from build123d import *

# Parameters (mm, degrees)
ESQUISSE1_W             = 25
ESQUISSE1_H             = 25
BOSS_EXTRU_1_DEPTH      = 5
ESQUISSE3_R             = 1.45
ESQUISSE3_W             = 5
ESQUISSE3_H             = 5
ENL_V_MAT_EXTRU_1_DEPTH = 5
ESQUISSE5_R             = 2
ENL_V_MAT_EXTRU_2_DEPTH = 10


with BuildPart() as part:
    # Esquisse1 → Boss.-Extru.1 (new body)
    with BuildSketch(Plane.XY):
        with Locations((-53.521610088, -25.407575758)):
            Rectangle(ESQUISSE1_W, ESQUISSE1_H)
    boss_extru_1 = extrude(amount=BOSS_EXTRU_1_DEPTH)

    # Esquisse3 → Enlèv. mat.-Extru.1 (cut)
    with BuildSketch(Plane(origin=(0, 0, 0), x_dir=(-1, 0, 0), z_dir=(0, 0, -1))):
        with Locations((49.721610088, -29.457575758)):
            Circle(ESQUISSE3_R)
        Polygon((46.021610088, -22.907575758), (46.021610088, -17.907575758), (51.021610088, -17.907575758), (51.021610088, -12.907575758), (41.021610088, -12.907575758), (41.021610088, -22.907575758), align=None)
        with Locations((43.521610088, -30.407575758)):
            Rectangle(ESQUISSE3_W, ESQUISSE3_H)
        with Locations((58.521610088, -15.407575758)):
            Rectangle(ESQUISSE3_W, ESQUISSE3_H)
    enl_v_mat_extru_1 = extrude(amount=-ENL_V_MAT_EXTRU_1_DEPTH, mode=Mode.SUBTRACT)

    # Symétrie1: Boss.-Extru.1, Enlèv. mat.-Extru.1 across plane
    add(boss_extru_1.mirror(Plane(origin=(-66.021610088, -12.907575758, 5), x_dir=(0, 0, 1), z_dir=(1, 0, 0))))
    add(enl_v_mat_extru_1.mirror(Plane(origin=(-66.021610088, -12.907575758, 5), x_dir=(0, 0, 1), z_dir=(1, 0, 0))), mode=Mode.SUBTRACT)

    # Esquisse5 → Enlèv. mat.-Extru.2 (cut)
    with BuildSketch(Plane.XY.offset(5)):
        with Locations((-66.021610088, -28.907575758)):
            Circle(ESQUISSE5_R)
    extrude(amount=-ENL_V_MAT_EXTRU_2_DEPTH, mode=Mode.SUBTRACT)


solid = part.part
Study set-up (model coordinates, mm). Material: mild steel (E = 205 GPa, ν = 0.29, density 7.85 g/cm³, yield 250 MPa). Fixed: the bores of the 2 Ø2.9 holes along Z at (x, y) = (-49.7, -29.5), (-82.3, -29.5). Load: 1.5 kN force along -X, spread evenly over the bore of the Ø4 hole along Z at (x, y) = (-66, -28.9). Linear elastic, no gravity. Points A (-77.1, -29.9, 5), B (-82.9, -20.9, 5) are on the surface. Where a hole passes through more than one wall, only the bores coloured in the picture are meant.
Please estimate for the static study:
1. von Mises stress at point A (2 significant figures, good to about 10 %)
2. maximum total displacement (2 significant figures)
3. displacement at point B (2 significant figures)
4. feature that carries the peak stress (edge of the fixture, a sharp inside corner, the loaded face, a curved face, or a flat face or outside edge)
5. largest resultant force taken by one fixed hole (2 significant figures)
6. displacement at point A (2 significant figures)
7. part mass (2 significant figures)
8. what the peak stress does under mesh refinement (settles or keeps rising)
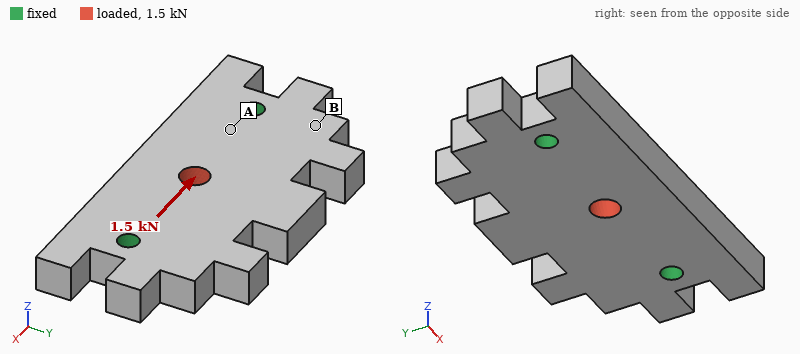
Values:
18 MPa
1.3 µm
0.57 µm
edge of the fixture
750 N
0.40 µm
38 g
keeps rising
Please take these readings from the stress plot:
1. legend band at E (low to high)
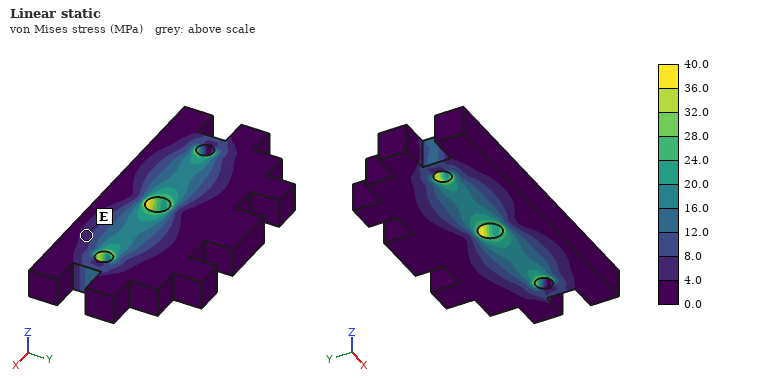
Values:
4.0 to 8.0 MPa
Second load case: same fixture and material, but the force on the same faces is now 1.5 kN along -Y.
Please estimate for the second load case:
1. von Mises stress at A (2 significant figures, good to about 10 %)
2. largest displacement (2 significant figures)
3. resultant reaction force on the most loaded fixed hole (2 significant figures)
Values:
17 MPa
3.2 µm
760 N
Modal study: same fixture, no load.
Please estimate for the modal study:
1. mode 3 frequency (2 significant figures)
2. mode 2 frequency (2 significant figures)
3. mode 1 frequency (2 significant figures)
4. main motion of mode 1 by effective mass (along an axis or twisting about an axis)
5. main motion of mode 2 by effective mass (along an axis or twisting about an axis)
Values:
22 kHz
20 kHz
12 kHz
along Z
along Z
